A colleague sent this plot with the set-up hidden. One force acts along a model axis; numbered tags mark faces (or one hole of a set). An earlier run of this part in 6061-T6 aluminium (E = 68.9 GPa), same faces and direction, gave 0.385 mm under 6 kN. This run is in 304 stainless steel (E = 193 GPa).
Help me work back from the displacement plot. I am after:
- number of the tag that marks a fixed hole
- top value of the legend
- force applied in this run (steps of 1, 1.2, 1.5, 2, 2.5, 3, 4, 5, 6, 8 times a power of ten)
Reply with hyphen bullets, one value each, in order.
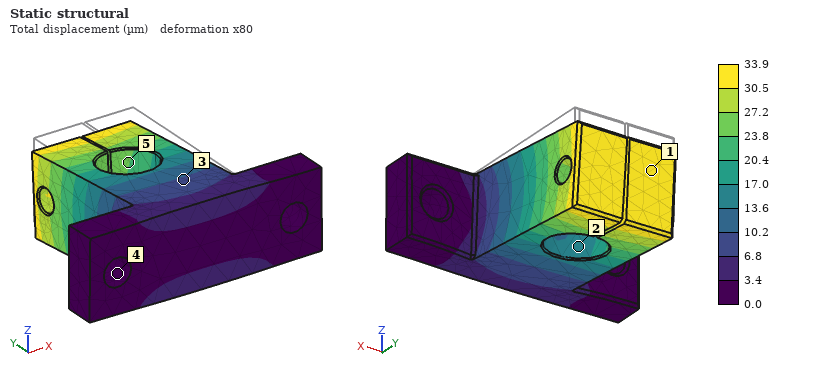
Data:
- 4
- 33.9 µm
- 1.5 kN
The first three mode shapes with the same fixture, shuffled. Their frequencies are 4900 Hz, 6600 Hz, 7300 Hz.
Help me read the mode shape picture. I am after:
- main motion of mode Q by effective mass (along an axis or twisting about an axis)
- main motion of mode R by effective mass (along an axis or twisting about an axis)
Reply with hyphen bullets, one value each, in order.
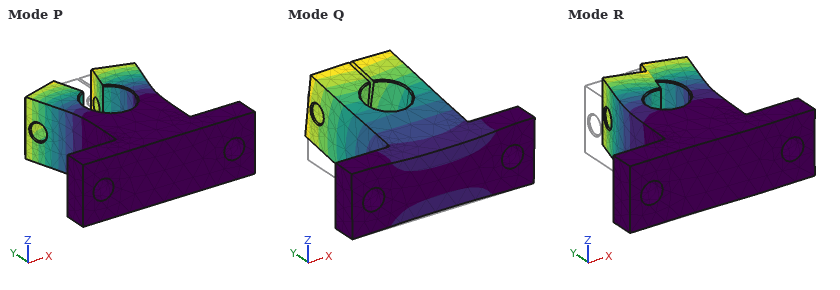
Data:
- along Z
- along X
